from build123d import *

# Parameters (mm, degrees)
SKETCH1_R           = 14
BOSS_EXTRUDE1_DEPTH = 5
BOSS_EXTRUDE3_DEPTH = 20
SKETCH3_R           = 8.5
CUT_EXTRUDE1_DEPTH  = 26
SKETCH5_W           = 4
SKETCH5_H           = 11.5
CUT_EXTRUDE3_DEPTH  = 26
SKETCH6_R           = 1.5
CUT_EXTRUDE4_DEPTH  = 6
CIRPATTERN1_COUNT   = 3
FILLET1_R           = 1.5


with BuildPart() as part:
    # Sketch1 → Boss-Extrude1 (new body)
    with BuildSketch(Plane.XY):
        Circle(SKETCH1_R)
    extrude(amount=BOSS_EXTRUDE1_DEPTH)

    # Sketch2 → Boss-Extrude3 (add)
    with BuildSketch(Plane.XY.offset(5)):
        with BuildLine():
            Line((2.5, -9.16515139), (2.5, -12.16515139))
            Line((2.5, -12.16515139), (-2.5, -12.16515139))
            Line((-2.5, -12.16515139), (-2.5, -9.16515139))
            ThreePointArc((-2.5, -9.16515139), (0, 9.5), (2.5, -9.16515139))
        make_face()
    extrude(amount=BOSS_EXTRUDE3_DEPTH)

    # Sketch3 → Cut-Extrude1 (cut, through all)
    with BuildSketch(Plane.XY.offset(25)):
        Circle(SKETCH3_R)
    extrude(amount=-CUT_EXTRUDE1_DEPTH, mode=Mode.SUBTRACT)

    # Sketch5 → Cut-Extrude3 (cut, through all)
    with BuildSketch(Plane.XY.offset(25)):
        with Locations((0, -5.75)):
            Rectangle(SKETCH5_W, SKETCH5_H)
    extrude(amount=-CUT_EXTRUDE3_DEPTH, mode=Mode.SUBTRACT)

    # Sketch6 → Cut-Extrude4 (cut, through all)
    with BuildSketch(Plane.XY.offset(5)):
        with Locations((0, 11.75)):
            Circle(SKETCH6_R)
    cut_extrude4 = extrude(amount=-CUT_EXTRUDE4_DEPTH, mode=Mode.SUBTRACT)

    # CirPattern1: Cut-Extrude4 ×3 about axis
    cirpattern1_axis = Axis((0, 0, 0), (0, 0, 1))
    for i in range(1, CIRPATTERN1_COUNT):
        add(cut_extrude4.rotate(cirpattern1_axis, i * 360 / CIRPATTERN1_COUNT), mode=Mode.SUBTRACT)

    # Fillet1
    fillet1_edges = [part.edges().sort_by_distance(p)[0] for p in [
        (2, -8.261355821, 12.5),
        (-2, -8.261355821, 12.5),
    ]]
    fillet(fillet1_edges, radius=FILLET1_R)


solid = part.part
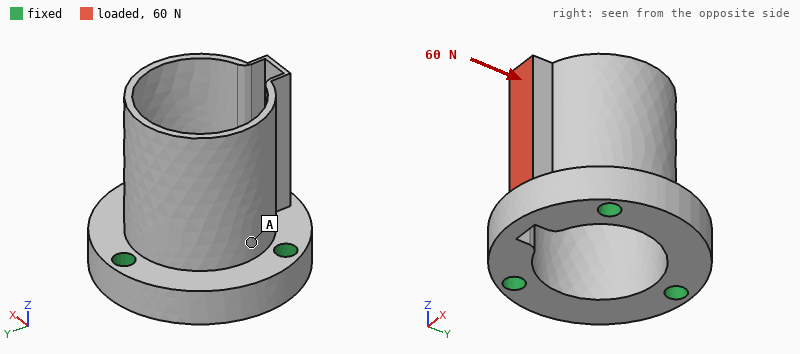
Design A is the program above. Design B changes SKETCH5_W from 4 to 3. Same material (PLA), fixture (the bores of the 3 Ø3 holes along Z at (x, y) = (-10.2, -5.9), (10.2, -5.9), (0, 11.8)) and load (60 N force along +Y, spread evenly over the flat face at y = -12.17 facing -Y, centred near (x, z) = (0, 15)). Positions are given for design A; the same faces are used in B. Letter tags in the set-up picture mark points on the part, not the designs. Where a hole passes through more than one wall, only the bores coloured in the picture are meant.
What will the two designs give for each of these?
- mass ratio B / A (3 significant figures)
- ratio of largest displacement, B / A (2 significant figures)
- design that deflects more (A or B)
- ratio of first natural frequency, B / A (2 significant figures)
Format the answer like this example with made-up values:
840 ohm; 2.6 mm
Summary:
1.03; 0.83; A; 1.2
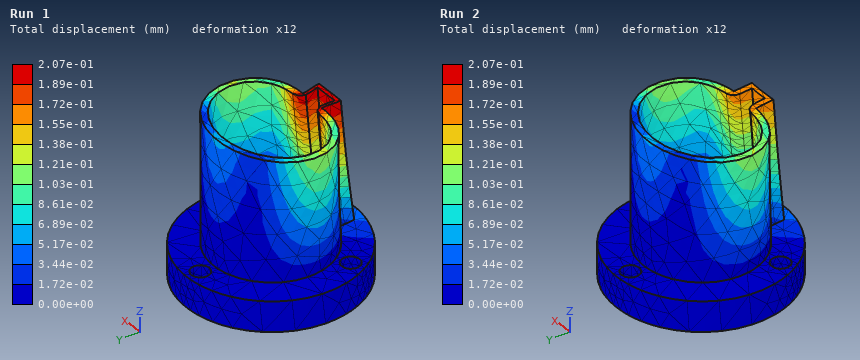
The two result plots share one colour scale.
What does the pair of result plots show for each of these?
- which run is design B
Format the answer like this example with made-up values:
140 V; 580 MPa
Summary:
Run 2
